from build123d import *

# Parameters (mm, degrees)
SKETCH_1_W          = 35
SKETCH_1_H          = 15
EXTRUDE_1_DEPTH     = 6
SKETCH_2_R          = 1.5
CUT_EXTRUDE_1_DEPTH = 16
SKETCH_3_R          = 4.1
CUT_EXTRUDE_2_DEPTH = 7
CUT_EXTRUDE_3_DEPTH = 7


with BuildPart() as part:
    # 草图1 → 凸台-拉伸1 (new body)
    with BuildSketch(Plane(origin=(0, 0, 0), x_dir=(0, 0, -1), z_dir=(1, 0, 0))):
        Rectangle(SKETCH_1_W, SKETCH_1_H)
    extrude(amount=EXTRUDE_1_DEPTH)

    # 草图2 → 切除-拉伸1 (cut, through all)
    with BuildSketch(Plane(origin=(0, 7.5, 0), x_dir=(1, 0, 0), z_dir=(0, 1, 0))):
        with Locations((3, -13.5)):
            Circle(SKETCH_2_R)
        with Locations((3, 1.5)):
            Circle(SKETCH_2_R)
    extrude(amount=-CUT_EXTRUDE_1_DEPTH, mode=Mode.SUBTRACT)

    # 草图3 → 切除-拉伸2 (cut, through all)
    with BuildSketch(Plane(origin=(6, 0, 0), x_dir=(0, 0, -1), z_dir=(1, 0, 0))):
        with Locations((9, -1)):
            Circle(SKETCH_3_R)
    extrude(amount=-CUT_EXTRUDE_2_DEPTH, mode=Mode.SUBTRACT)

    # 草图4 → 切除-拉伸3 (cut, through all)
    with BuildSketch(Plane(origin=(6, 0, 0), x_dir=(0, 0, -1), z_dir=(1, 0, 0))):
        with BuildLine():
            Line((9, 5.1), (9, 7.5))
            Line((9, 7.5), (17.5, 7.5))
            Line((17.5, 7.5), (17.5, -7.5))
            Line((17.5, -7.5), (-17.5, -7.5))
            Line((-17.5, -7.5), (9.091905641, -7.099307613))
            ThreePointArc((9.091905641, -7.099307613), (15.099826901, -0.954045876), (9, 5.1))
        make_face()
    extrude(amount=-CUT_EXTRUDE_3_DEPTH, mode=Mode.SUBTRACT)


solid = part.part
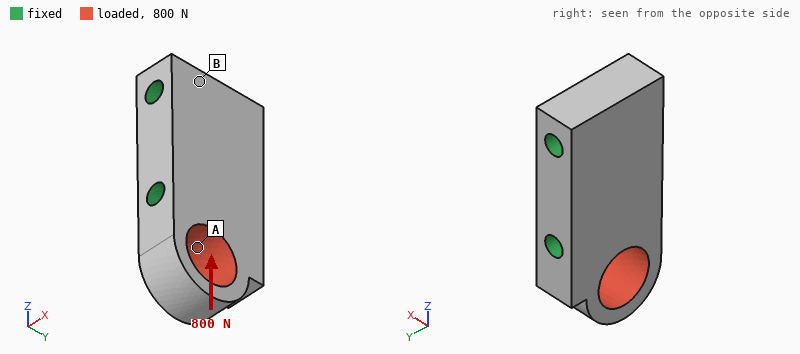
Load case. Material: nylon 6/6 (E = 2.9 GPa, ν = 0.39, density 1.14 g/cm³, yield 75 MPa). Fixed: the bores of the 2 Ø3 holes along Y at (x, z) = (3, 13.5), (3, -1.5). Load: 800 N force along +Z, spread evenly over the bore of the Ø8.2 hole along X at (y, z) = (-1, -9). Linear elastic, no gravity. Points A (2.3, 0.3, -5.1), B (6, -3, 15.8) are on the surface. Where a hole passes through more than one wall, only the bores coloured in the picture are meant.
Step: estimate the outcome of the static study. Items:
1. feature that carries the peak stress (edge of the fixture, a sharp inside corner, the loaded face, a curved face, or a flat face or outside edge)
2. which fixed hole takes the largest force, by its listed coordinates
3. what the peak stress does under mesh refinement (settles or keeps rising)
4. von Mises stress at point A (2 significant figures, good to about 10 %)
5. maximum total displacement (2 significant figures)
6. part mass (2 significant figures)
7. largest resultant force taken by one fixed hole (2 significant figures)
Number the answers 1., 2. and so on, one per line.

1. edge of the fixture
2. (3, -1.5)
3. keeps rising
4. 8.0 MPa
5. 0.14 mm
6. 2.5 g
7. 780 N
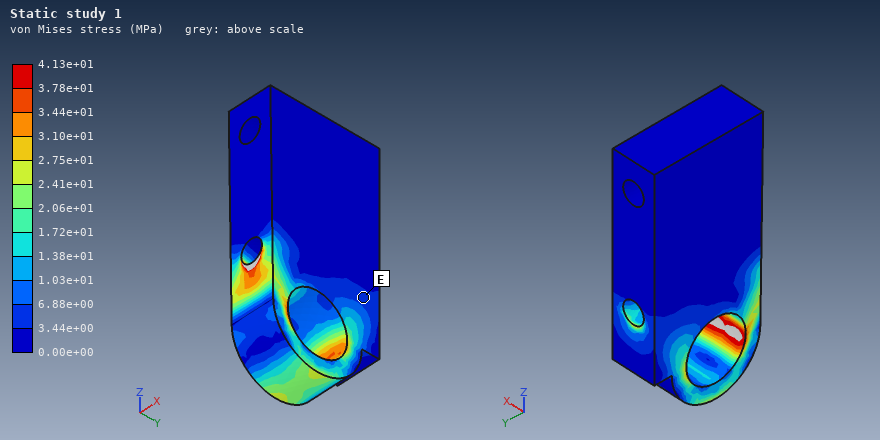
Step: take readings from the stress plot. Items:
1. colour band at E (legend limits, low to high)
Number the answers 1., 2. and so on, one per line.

1. 3.44e+00 to 6.88e+00 MPa
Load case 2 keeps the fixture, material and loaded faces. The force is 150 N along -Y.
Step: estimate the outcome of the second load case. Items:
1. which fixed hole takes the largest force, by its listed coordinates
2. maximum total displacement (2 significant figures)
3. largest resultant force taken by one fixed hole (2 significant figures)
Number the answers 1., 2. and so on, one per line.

1. (3, -1.5)
2. 92 µm
3. 150 N
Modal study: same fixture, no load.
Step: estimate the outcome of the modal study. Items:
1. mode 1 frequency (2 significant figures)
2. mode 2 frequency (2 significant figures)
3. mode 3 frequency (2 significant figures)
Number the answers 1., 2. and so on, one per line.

1. 8500 Hz
2. 11 kHz
3. 15 kHz
